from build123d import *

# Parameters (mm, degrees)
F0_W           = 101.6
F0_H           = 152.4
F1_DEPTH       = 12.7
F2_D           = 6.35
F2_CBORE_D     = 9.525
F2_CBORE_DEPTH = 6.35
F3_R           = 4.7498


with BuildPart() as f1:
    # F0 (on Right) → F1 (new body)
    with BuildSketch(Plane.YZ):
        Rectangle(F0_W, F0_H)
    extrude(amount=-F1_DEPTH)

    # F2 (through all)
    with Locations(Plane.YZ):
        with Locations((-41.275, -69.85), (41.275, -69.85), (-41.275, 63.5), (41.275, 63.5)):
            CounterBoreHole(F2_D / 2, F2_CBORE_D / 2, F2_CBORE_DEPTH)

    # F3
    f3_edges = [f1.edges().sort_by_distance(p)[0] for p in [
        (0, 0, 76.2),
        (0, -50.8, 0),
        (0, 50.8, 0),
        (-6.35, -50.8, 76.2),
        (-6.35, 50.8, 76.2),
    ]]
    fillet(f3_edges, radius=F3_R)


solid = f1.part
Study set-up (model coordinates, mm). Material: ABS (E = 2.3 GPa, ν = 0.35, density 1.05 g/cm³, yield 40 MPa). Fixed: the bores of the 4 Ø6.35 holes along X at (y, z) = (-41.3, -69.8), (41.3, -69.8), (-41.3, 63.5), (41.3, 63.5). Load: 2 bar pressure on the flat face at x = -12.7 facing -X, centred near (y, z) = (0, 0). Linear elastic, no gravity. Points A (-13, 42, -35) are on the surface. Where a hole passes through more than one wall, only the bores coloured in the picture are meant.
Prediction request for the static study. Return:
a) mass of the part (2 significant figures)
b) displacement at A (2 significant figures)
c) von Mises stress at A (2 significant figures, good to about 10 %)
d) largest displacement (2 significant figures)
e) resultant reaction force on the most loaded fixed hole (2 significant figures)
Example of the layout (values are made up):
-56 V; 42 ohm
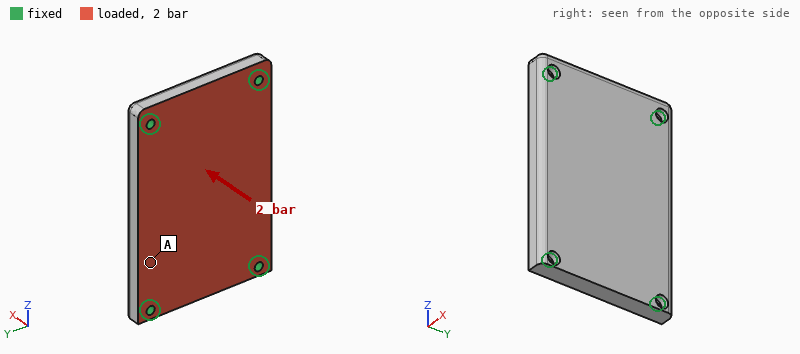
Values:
200 g; 0.70 mm; 4.7 MPa; 1.0 mm; 1.1 kN
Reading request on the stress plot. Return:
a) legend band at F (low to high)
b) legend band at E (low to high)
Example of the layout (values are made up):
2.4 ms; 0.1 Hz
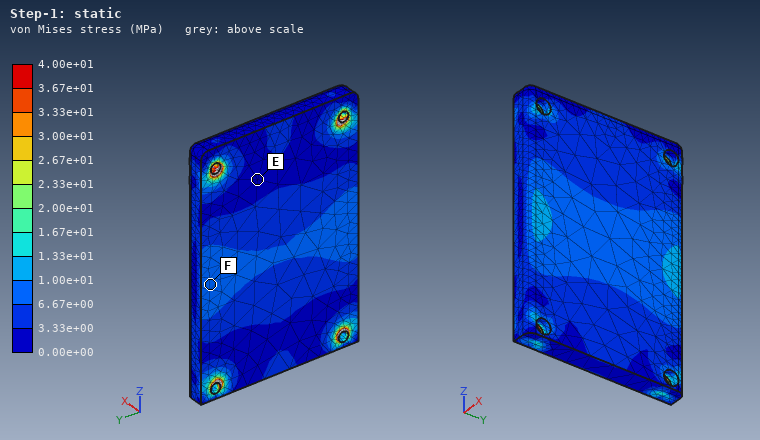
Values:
6.67e+00 to 1.00e+01 MPa; 0.00e+00 to 3.33e+00 MPa
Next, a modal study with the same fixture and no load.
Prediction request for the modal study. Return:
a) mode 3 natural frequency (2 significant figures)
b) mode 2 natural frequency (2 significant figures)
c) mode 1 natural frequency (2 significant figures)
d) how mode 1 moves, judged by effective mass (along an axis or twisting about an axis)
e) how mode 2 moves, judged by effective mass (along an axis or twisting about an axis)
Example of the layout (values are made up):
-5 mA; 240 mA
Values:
1700 Hz; 1100 Hz; 690 Hz; along X; twisting about Z
